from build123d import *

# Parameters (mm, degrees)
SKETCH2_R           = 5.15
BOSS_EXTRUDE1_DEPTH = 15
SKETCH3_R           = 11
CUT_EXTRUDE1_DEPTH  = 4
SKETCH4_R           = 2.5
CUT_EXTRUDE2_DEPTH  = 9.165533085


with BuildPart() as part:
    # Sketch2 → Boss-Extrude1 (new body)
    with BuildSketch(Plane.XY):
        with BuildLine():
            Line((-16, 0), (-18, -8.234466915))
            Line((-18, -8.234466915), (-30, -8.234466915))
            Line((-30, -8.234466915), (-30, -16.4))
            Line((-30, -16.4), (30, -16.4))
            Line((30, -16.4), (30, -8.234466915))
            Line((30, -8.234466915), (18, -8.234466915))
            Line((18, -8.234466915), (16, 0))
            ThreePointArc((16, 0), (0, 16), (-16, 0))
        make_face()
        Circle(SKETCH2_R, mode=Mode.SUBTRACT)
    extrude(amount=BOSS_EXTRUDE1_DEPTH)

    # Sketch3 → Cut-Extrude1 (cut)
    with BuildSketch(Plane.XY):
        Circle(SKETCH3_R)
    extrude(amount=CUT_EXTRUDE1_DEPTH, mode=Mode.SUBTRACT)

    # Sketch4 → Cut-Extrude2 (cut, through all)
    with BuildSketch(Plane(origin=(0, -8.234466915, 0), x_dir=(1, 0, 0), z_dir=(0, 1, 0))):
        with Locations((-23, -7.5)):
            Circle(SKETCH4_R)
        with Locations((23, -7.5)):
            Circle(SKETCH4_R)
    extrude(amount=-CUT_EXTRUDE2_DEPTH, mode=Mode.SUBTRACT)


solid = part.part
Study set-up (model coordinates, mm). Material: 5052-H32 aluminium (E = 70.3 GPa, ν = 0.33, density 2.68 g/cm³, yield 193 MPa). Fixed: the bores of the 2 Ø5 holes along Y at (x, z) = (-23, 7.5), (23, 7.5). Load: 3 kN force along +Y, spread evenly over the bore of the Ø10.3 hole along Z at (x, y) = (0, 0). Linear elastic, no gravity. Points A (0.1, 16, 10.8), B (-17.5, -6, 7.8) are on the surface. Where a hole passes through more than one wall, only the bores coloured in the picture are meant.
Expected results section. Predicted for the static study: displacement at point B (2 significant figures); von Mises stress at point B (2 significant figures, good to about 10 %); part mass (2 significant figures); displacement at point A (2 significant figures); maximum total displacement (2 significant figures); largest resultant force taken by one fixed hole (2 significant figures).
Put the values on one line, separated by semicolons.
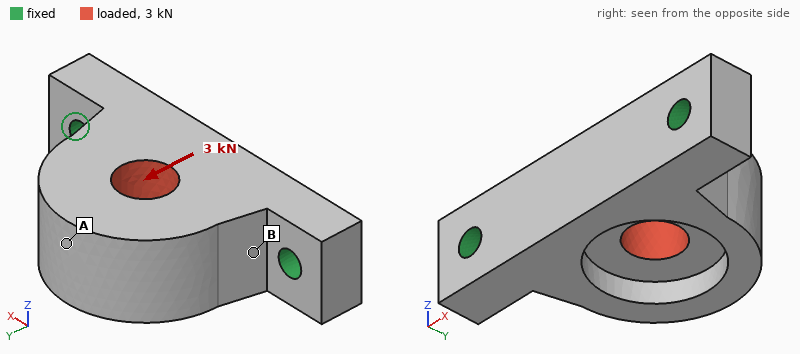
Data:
5.8 µm; 30 MPa; 40 g; 18 µm; 20 µm; 1.6 kN
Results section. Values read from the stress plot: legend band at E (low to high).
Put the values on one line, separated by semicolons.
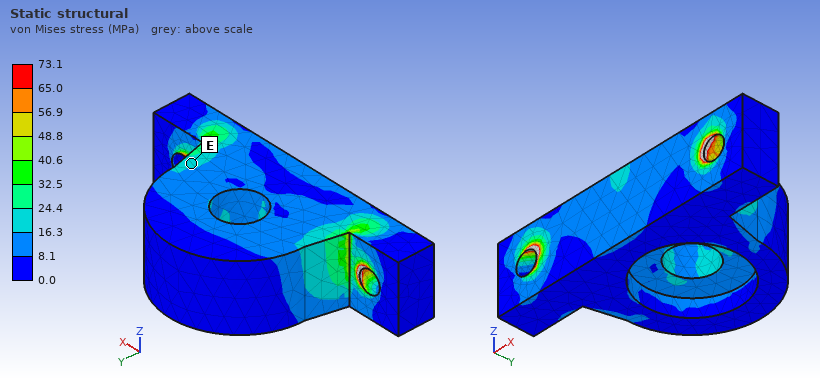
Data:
16.3 to 24.4 MPa
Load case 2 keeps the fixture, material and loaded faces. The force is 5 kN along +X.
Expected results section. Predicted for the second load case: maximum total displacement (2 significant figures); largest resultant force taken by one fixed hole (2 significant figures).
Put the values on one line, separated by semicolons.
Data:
16 µm; 2.9 kN
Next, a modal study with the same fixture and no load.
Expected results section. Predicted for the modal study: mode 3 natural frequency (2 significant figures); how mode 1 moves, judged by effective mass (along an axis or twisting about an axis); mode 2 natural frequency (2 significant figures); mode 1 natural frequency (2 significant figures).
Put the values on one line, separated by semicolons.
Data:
18 kHz; along Z; 18 kHz; 6600 Hz
